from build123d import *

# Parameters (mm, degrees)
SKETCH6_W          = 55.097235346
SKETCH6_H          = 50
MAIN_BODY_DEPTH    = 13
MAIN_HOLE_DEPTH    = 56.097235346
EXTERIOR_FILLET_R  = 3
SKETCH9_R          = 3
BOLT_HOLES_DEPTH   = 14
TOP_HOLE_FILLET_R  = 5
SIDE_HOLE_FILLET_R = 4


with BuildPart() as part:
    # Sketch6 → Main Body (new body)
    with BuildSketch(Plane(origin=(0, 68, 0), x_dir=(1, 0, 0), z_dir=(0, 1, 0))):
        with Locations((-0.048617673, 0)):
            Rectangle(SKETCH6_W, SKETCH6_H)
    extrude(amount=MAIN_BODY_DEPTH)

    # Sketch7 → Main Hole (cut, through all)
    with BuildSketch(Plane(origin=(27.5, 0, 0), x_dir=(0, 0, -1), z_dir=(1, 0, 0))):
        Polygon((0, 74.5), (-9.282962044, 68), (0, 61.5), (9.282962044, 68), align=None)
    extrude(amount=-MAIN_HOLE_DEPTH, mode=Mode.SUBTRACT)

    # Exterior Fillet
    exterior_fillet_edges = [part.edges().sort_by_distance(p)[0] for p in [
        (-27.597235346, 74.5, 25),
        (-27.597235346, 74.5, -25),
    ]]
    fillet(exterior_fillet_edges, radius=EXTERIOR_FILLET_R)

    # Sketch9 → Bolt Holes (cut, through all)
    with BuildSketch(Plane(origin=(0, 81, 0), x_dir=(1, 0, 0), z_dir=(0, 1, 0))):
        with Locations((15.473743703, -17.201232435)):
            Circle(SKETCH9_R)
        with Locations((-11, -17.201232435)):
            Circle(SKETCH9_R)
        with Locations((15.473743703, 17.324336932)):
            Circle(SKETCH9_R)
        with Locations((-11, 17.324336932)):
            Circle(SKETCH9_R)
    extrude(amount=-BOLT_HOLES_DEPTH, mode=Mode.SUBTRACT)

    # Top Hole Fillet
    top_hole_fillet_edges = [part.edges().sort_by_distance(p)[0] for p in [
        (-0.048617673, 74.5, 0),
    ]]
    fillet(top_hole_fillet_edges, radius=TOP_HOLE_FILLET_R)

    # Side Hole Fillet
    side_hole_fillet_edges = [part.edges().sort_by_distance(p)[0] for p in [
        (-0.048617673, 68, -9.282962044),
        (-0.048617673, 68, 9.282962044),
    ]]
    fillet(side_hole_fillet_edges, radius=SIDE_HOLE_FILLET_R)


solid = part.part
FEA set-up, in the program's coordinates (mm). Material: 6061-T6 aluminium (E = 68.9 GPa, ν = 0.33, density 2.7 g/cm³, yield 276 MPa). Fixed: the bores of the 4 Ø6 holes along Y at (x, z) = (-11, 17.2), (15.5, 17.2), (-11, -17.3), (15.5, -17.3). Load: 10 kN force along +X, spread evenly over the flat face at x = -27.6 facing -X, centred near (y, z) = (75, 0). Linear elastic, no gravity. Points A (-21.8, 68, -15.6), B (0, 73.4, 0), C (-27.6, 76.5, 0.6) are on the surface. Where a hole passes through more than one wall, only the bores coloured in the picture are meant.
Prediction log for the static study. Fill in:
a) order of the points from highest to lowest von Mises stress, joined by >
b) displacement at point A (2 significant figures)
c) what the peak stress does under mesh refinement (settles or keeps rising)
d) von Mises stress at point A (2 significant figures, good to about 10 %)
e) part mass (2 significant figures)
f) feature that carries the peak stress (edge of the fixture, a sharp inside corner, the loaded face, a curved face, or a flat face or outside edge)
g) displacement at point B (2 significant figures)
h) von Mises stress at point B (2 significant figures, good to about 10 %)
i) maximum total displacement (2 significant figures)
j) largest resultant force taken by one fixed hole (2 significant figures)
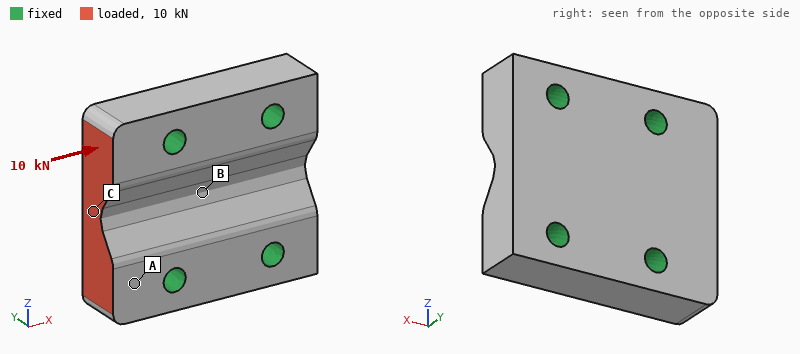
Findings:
A > C > B
3.1 µm
keeps rising
22 MPa
84 g
edge of the fixture
1.6 µm
6.9 MPa
7.7 µm
4.3 kN
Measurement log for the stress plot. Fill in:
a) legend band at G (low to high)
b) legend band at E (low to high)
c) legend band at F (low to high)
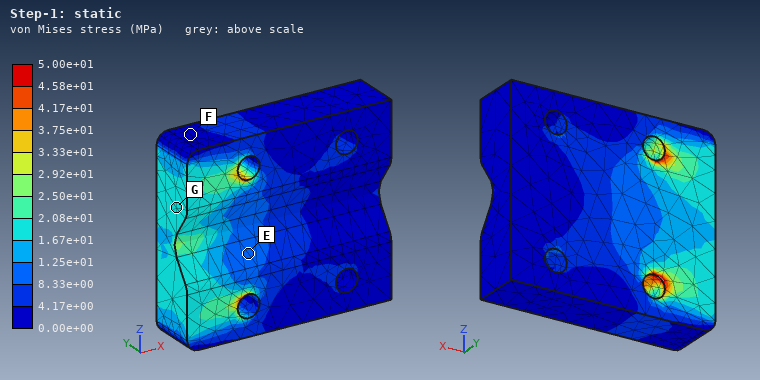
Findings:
1.67e+01 to 2.08e+01 MPa
8.33e+00 to 1.25e+01 MPa
0.00e+00 to 4.17e+00 MPa
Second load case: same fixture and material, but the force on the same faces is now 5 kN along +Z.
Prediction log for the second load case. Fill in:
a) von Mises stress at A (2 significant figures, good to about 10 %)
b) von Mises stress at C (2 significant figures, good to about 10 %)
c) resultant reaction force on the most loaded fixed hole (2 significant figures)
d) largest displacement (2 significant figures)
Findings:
13 MPa
20 MPa
3.1 kN
9.5 µm
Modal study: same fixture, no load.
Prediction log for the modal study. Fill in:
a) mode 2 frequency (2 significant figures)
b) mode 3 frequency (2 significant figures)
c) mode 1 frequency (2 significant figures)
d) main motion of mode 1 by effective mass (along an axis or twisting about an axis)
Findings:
33 kHz
33 kHz
25 kHz
along Y
